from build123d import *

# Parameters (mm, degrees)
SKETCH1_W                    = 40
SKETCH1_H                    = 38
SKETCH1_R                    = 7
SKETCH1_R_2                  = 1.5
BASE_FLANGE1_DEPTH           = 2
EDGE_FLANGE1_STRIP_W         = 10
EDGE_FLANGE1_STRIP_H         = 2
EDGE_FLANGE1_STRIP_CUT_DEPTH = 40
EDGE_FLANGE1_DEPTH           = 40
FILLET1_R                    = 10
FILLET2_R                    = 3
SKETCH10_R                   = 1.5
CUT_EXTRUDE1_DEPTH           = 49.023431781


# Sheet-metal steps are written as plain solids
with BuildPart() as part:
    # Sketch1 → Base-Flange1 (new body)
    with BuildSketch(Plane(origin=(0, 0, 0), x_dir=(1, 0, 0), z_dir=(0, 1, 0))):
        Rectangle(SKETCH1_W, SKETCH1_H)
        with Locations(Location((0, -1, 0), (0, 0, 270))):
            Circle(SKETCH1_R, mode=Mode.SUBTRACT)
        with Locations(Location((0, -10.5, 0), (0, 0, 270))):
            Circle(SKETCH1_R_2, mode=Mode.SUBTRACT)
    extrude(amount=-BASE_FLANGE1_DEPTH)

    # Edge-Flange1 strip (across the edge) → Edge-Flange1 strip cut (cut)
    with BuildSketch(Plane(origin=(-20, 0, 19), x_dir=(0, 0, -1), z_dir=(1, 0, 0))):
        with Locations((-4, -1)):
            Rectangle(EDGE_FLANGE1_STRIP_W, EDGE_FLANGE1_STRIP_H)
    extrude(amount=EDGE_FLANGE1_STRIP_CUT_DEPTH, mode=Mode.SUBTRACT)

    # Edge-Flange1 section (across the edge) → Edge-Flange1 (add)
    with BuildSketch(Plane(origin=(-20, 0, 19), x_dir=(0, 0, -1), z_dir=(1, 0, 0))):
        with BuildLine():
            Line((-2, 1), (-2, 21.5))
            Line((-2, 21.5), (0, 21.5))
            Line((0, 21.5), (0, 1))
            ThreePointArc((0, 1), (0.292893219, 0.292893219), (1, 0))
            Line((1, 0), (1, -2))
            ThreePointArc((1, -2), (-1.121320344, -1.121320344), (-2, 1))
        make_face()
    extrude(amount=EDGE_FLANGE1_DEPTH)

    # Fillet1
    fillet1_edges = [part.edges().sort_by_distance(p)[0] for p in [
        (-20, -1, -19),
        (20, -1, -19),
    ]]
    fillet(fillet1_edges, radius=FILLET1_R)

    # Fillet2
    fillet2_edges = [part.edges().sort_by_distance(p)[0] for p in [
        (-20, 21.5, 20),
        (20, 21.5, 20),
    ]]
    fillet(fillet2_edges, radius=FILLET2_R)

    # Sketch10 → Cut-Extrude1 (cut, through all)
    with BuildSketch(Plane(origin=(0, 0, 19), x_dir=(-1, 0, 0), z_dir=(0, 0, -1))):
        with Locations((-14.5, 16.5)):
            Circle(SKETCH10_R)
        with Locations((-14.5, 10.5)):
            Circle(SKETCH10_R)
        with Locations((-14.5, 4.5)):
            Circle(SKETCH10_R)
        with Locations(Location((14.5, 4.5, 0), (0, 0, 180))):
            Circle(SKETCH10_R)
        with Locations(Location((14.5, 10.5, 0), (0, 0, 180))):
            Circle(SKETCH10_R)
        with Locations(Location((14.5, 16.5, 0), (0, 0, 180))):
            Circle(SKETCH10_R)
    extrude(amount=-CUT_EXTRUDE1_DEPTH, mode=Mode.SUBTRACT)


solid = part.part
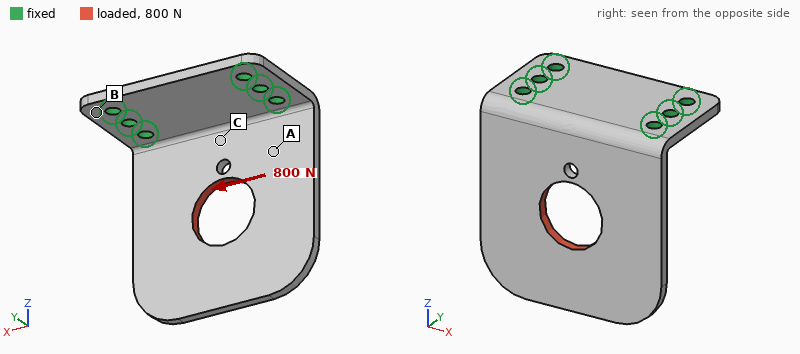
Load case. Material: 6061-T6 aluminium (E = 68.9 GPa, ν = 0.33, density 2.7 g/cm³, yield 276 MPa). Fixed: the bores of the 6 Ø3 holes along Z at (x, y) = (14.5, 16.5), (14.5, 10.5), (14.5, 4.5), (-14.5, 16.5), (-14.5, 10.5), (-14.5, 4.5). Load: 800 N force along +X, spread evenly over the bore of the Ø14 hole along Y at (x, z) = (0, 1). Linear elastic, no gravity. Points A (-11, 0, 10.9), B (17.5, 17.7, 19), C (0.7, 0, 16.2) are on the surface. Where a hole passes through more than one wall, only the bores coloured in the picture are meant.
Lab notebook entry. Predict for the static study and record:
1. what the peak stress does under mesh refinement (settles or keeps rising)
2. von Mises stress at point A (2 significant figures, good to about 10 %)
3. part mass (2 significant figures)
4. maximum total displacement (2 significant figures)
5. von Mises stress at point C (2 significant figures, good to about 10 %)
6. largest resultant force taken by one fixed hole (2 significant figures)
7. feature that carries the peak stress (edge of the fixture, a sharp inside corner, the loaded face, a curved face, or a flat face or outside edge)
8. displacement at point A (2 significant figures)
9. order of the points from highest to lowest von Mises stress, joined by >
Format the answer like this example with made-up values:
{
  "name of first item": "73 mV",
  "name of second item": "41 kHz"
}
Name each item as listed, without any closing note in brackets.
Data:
{
  "what the peak stress does under mesh refinement": "keeps rising",
  "von Mises stress at point A": "41 MPa",
  "part mass": "12 g",
  "maximum total displacement": "0.15 mm",
  "von Mises stress at point C": "69 MPa",
  "largest resultant force taken by one fixed hole": "660 N",
  "feature that carries the peak stress": "edge of the fixture",
  "displacement at point A": "0.049 mm",
  "order of the points from highest to lowest von Mises stress, joined by >": "C > A > B"
}
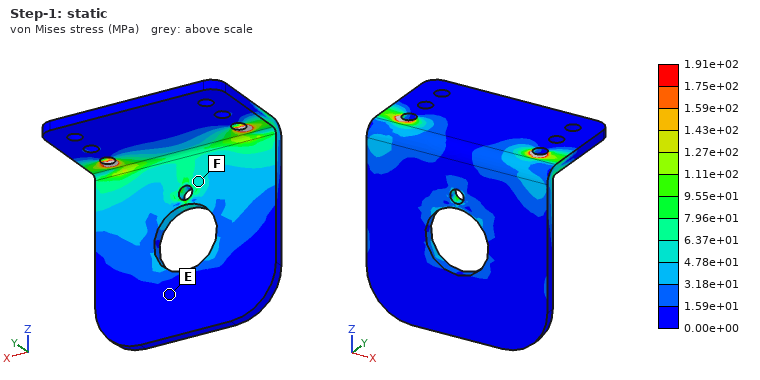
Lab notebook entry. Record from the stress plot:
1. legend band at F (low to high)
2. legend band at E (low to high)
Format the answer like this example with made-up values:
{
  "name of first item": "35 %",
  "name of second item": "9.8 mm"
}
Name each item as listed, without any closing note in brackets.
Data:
{
  "legend band at F": "4.78e+01 to 6.37e+01 MPa",
  "legend band at E": "0.00e+00 to 1.59e+01 MPa"
}
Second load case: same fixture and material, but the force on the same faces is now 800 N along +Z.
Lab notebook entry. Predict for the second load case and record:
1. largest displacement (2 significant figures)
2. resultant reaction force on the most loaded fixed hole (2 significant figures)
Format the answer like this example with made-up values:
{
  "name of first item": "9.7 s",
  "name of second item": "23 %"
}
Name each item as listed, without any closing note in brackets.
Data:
{
  "largest displacement": "0.26 mm",
  "resultant reaction force on the most loaded fixed hole": "490 N"
}
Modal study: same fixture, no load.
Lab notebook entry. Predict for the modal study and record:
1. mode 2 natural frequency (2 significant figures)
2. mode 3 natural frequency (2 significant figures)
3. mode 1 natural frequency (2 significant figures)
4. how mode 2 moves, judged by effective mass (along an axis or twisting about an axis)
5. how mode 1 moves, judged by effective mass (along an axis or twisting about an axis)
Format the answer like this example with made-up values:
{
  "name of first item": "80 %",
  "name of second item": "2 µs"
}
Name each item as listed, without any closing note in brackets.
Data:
{
  "mode 2 natural frequency": "2400 Hz",
  "mode 3 natural frequency": "5400 Hz",
  "mode 1 natural frequency": "930 Hz",
  "how mode 2 moves, judged by effective mass": "twisting about Z",
  "how mode 1 moves, judged by effective mass": "along Y"
}
